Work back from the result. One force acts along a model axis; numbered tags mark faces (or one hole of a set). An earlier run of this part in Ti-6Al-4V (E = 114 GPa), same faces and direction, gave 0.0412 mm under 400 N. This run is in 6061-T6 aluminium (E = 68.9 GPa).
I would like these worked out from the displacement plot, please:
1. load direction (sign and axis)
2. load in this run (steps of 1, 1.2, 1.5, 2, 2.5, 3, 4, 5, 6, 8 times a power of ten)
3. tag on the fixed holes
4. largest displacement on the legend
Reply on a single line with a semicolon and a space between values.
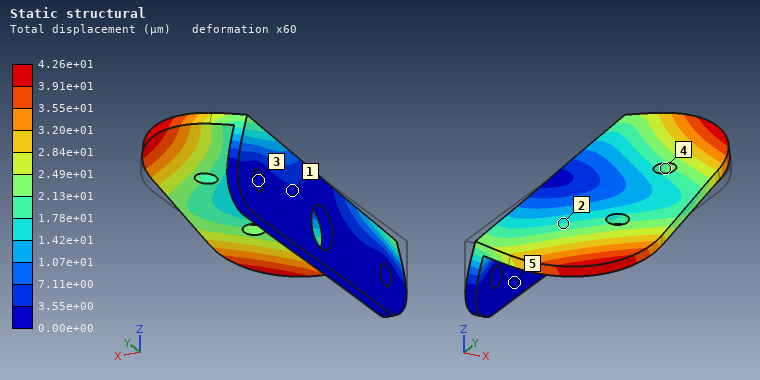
+Y; 250 N; 3; 4.26e+01 µm
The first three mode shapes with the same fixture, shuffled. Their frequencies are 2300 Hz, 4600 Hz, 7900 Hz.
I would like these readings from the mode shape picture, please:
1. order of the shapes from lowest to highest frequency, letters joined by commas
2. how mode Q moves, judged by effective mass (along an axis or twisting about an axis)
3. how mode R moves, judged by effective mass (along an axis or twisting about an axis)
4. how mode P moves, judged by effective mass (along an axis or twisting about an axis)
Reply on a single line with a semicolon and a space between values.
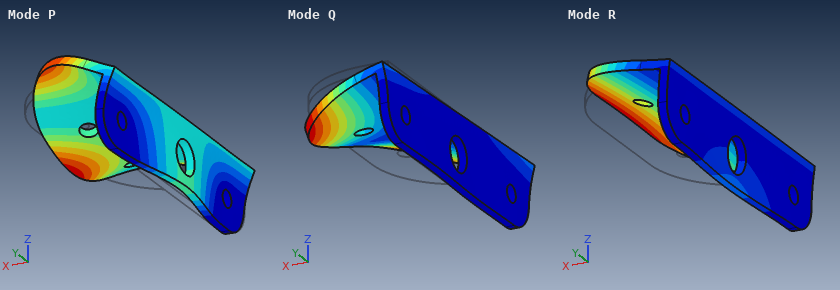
R, Q, P; twisting about X; along Z; along X
